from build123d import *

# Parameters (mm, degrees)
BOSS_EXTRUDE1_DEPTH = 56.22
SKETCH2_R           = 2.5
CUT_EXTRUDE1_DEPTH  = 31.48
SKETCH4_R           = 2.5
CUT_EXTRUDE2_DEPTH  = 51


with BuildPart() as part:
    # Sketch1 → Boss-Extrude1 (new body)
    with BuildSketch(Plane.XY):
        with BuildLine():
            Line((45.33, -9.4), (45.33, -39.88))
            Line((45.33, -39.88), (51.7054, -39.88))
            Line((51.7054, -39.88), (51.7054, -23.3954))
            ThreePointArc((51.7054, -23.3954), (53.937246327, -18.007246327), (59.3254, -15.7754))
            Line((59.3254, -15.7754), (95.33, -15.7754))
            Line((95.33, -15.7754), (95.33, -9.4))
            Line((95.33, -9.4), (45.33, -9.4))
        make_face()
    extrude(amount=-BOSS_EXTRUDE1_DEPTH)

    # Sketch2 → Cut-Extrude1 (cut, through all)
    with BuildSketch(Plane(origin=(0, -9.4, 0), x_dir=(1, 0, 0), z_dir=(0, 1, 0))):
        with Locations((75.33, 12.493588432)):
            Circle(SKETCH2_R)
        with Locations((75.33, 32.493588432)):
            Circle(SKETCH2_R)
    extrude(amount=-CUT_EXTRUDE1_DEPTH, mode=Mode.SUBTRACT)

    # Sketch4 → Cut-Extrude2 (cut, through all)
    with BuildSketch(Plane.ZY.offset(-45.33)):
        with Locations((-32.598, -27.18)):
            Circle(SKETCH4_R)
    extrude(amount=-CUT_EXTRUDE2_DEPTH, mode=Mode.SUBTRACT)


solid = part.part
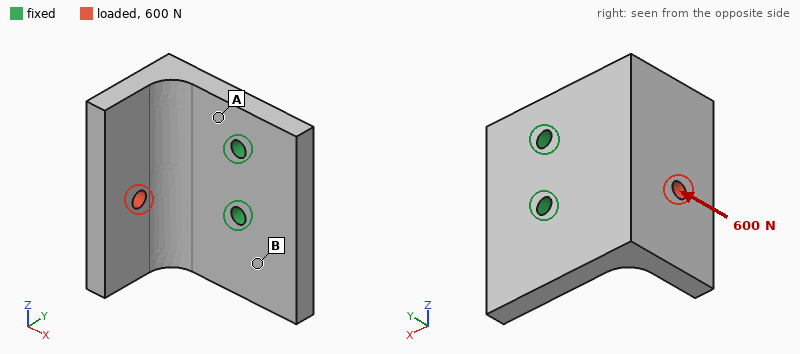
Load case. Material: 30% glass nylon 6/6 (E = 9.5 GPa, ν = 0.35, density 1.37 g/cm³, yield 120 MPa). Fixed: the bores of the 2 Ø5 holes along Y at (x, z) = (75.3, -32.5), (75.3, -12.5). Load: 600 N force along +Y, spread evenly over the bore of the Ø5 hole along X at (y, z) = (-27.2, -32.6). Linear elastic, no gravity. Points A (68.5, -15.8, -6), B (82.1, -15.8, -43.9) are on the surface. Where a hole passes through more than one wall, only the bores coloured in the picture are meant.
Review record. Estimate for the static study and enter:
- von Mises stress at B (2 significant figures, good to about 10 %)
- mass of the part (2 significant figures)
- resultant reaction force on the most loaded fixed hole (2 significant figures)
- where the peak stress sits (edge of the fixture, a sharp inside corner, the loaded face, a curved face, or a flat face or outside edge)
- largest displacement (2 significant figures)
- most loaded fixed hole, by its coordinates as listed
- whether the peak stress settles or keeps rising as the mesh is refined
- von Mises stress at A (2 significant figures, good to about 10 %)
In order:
11 MPa
37 g
500 N
edge of the fixture
0.80 mm
(75.3, -32.5)
keeps rising
25 MPa
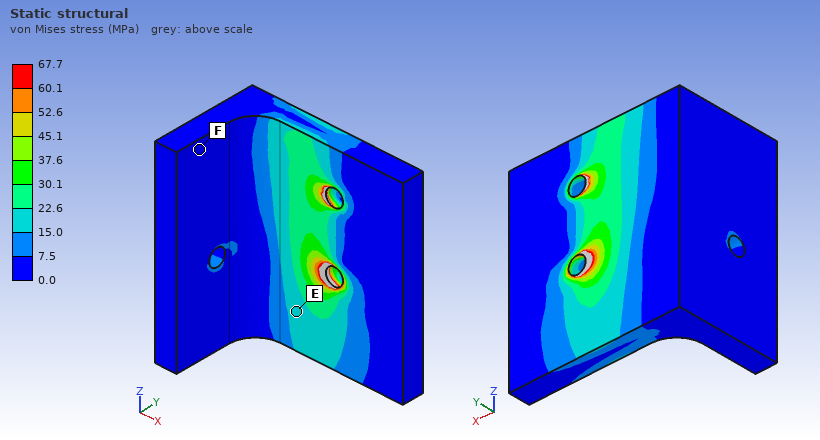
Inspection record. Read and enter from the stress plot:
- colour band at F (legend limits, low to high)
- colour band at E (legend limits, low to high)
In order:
0.0 to 7.5 MPa
15.0 to 22.6 MPa
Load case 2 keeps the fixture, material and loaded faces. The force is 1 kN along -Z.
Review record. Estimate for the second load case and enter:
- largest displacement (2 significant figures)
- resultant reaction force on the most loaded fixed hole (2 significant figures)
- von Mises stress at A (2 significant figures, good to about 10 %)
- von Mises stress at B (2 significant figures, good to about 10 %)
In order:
0.49 mm
1.3 kN
17 MPa
8.8 MPa
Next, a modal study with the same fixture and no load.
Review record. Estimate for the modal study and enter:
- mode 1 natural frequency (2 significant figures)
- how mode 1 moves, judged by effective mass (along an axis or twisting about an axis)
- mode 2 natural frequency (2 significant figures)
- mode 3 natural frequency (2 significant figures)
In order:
1200 Hz
along Y
2000 Hz
3900 Hz
